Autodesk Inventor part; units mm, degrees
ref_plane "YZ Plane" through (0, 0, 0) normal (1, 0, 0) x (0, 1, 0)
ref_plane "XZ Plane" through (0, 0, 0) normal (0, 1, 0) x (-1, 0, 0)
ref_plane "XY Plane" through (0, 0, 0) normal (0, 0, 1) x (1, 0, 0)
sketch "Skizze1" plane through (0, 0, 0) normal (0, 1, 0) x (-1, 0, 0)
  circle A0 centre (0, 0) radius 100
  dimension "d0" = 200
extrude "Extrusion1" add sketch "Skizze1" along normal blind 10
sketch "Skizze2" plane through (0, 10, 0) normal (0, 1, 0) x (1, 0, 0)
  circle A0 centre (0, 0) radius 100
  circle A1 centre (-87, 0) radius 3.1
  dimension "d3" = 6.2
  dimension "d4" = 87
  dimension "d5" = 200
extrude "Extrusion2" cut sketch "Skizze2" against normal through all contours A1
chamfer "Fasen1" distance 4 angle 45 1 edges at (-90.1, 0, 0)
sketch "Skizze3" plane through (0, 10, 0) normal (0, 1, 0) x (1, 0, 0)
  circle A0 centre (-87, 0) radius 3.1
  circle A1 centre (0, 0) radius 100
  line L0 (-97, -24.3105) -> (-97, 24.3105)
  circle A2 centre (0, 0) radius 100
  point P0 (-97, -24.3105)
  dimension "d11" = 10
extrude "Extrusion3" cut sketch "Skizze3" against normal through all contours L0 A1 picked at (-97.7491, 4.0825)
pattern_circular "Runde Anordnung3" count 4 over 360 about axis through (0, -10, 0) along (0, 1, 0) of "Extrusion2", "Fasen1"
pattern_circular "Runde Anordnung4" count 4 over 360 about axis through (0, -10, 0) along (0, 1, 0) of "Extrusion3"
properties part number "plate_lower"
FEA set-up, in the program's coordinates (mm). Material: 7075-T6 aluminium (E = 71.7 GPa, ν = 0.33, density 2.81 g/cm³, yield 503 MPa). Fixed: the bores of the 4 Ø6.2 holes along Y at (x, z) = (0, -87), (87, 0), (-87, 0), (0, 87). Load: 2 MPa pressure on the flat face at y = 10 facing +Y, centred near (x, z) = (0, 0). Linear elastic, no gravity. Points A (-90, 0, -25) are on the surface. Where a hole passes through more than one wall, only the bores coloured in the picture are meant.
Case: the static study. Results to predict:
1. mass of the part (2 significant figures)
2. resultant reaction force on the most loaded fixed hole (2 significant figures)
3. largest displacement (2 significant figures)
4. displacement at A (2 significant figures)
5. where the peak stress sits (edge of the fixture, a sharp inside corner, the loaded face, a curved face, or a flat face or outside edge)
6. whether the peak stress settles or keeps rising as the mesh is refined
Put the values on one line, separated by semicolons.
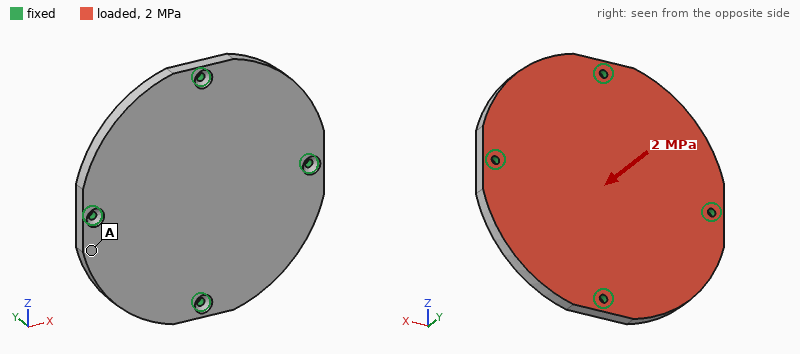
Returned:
870 g; 17 kN; 0.70 mm; 0.11 mm; edge of the fixture; keeps rising
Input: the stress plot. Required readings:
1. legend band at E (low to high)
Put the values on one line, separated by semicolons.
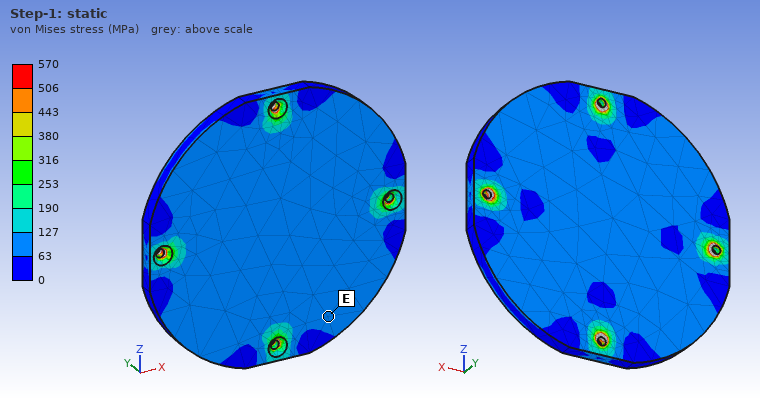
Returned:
63 to 127 MPa
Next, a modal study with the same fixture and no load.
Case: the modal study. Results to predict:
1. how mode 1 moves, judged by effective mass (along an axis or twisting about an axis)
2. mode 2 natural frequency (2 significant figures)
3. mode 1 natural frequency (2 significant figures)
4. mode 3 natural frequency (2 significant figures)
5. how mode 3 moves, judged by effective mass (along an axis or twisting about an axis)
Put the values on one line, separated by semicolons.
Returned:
along Y; 2100 Hz; 1900 Hz; 2300 Hz; twisting about Z
